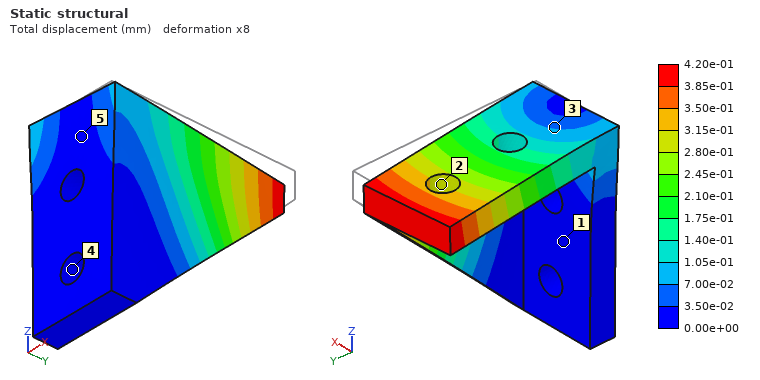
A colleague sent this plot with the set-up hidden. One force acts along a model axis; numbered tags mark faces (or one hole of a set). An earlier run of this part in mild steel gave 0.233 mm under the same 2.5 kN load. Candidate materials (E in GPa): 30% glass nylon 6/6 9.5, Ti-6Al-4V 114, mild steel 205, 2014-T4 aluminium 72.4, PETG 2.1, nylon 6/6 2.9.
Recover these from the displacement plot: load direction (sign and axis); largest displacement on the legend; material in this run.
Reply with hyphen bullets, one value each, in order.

- -X
- 4.20e-01 mm
- Ti-6Al-4V
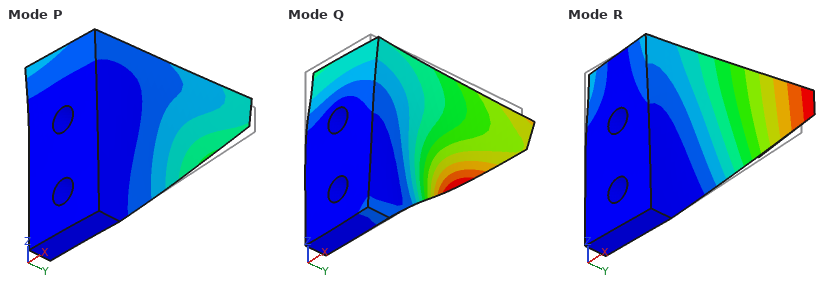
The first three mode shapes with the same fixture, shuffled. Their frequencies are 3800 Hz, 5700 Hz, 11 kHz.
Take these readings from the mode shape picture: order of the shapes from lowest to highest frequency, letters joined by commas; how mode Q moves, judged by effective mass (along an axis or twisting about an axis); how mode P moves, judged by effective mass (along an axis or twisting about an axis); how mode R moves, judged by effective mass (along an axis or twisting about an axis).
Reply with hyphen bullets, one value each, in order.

- R, P, Q
- along Y
- along Z
- along X
